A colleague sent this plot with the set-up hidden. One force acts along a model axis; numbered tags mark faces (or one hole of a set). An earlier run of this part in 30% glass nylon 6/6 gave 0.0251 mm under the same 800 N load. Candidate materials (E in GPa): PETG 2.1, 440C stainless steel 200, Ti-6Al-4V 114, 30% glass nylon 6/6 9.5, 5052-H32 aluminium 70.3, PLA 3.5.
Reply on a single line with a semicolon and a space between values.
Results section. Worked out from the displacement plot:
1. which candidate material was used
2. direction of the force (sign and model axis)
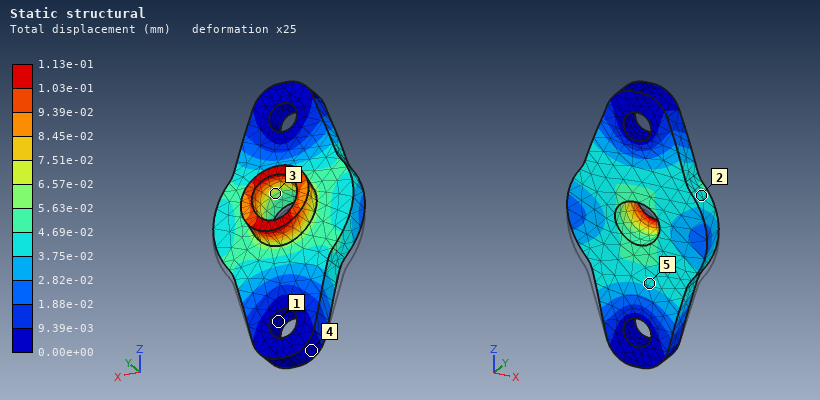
PETG; +Z
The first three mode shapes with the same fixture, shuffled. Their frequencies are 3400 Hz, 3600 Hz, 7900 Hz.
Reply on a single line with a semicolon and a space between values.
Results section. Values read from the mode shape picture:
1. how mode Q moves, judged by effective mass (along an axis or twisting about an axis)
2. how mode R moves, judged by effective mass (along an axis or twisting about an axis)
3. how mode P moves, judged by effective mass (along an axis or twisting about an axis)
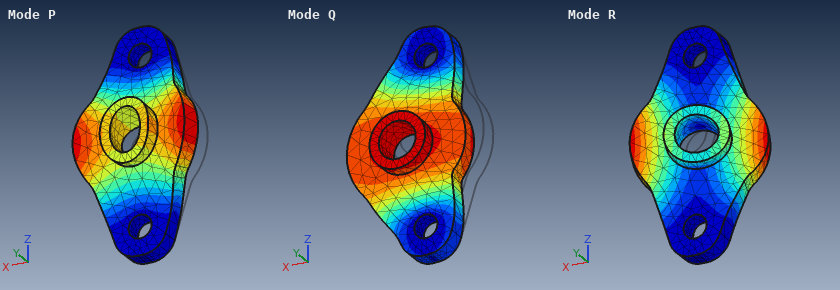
along X; twisting about Z; along Y
